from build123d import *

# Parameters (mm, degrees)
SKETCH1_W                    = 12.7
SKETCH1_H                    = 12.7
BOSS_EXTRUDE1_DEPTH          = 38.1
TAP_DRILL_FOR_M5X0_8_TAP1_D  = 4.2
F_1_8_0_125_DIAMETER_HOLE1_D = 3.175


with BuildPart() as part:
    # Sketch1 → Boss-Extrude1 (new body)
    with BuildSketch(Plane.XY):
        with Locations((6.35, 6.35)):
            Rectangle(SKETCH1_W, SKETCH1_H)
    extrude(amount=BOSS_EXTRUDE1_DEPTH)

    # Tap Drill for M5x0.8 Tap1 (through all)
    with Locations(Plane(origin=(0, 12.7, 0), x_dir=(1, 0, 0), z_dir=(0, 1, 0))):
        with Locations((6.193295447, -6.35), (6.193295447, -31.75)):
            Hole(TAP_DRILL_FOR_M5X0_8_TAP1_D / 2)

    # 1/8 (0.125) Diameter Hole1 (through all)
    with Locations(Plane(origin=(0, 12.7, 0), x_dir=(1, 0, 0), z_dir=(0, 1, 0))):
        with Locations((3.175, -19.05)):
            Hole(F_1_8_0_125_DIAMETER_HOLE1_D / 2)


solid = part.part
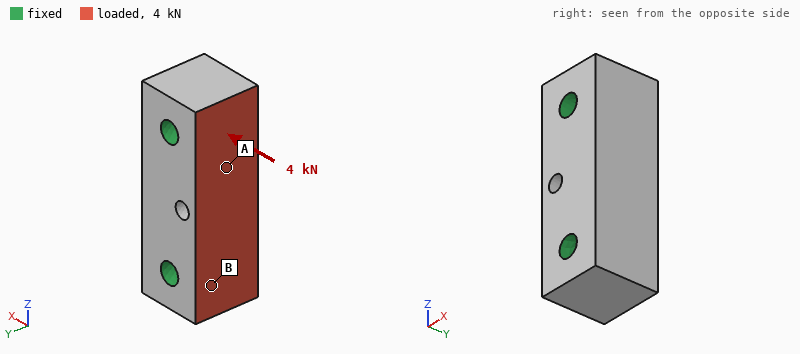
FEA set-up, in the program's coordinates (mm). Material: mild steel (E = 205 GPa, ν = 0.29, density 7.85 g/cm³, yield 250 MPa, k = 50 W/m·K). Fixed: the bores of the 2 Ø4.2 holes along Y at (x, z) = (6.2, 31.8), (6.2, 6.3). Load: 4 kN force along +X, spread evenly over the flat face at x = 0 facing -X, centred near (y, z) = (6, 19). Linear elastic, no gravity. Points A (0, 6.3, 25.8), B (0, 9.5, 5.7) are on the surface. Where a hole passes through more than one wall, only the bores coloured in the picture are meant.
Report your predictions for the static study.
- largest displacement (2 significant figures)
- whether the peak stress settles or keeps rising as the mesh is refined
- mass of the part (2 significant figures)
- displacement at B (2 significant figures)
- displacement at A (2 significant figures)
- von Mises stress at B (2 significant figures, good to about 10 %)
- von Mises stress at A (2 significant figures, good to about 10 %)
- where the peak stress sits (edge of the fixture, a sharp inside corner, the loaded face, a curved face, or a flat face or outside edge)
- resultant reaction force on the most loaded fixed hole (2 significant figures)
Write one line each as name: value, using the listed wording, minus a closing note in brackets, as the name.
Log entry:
largest displacement: 1.4 µm
whether the peak stress settles or keeps rising as the mesh is refined: keeps rising
mass of the part: 45 g
displacement at B: 0.26 µm
displacement at A: 0.85 µm
von Mises stress at B: 15 MPa
von Mises stress at A: 7.3 MPa
where the peak stress sits: edge of the fixture
resultant reaction force on the most loaded fixed hole: 2.0 kN
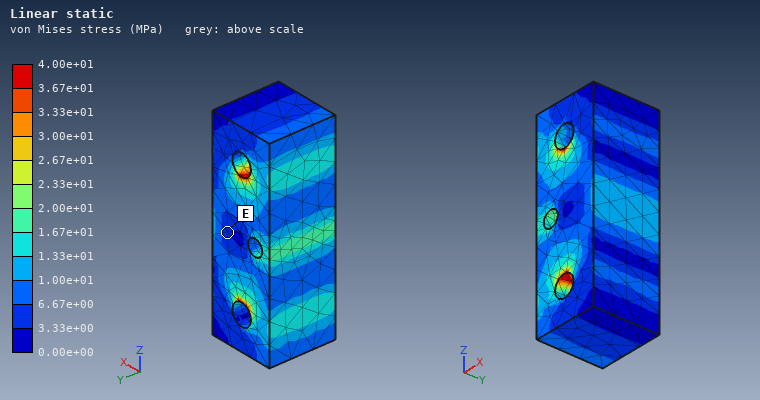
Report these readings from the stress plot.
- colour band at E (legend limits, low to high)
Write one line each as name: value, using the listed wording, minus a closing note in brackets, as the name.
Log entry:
colour band at E: 3.33e+00 to 6.67e+00 MPa
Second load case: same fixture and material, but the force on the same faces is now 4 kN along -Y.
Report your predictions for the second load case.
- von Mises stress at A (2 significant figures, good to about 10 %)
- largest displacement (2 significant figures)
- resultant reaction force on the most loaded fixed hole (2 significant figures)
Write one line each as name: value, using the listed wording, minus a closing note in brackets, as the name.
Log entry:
von Mises stress at A: 30 MPa
largest displacement: 3.3 µm
resultant reaction force on the most loaded fixed hole: 2.0 kN
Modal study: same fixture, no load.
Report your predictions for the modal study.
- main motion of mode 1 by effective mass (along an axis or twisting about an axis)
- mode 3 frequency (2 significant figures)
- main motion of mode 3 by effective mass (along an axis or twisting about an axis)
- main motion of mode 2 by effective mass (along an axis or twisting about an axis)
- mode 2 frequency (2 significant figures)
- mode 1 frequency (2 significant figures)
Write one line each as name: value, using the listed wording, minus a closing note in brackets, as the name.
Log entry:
main motion of mode 1 by effective mass: along X
mode 3 frequency: 61 kHz
main motion of mode 3 by effective mass: twisting about Z
main motion of mode 2 by effective mass: along Y
mode 2 frequency: 53 kHz
mode 1 frequency: 47 kHz
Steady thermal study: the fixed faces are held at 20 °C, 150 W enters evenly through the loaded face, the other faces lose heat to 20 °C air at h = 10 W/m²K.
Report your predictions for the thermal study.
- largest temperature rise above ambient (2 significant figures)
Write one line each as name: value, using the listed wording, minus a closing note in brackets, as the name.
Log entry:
largest temperature rise above ambient: 73 K
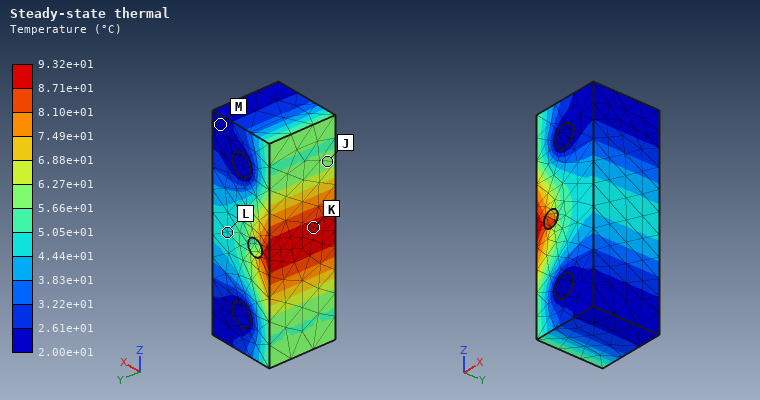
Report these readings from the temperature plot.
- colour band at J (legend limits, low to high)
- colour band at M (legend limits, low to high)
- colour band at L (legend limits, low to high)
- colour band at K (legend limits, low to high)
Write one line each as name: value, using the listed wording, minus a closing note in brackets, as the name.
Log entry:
colour band at J: 5.66e+01 to 6.27e+01 °C
colour band at M: 2.00e+01 to 2.61e+01 °C
colour band at L: 4.44e+01 to 5.05e+01 °C
colour band at K: 8.71e+01 to 9.32e+01 °C
